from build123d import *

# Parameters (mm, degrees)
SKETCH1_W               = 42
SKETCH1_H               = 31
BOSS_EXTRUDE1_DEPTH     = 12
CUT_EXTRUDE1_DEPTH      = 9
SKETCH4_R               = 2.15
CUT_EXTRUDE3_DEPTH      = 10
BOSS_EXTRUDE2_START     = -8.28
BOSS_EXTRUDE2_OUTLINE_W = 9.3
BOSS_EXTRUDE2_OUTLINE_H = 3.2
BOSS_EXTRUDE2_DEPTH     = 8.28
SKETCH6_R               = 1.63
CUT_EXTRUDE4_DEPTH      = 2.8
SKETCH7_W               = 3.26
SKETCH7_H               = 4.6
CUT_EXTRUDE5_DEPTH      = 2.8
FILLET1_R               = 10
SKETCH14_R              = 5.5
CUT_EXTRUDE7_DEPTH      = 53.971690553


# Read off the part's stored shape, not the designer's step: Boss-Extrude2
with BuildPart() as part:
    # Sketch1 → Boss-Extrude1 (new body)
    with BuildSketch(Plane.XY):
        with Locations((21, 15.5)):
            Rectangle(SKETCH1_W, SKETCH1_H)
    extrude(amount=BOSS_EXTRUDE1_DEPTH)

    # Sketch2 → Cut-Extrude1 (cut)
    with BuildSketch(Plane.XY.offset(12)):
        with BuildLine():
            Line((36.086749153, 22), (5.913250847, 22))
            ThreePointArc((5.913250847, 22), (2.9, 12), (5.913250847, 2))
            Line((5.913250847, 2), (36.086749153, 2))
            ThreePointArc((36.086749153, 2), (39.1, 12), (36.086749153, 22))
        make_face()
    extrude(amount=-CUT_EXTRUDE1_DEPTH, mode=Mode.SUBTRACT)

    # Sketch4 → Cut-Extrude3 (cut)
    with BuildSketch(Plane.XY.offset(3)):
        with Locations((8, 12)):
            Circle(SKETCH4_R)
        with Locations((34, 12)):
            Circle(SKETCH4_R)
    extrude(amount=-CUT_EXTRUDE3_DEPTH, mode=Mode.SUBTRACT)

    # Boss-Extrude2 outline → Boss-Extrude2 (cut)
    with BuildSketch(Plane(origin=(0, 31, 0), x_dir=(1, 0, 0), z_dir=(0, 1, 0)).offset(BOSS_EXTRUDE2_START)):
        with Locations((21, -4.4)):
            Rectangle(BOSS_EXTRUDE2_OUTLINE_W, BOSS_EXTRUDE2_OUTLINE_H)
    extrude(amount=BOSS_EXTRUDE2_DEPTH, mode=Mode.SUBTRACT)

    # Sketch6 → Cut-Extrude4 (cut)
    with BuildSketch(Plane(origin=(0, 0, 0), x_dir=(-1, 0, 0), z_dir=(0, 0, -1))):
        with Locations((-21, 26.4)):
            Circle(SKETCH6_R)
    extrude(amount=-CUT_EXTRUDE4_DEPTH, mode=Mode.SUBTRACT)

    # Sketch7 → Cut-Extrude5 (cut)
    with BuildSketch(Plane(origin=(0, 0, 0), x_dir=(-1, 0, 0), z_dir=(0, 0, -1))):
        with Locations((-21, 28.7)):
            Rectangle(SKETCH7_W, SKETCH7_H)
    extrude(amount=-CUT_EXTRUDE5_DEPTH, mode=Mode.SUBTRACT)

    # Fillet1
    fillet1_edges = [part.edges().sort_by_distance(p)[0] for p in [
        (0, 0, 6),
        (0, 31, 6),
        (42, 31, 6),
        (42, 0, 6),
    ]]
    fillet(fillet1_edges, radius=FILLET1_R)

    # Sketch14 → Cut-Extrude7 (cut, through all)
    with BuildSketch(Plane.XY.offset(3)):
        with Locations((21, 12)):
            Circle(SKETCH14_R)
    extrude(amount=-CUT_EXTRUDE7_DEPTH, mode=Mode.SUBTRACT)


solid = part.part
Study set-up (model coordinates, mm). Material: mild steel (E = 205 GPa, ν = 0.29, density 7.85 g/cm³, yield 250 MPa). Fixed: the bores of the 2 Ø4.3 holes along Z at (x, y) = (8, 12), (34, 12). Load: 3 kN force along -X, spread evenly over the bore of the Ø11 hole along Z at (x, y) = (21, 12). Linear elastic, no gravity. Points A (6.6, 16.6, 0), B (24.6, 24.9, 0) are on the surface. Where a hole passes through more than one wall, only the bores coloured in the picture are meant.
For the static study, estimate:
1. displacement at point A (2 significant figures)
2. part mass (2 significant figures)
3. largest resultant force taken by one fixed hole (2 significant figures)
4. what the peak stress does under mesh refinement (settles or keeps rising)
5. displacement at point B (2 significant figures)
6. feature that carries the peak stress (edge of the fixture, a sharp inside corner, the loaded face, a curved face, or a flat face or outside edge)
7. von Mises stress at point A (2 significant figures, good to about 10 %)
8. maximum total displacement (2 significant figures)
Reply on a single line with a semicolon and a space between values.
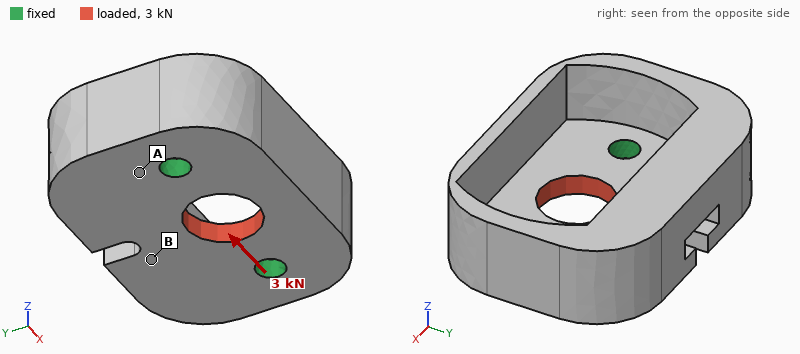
0.54 µm; 61 g; 1.5 kN; keeps rising; 1.2 µm; edge of the fixture; 19 MPa; 2.4 µm
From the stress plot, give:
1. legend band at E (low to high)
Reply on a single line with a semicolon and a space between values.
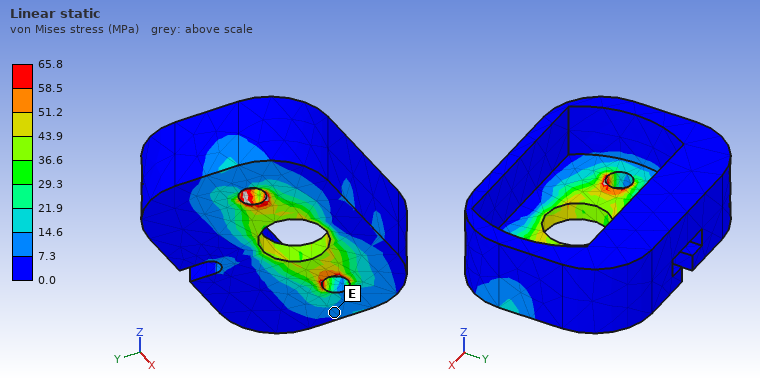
7.3 to 14.6 MPa
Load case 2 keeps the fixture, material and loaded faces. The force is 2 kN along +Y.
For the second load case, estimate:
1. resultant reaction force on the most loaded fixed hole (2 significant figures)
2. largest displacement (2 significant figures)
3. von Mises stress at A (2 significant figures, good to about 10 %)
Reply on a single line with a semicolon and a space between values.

1.0 kN; 2.7 µm; 13 MPa
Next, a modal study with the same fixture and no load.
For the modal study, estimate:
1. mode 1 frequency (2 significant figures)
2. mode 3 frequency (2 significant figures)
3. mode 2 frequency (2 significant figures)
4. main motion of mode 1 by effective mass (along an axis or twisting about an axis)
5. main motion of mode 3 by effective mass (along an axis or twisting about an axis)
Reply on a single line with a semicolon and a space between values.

5100 Hz; 14 kHz; 10 kHz; along Z; along Z
